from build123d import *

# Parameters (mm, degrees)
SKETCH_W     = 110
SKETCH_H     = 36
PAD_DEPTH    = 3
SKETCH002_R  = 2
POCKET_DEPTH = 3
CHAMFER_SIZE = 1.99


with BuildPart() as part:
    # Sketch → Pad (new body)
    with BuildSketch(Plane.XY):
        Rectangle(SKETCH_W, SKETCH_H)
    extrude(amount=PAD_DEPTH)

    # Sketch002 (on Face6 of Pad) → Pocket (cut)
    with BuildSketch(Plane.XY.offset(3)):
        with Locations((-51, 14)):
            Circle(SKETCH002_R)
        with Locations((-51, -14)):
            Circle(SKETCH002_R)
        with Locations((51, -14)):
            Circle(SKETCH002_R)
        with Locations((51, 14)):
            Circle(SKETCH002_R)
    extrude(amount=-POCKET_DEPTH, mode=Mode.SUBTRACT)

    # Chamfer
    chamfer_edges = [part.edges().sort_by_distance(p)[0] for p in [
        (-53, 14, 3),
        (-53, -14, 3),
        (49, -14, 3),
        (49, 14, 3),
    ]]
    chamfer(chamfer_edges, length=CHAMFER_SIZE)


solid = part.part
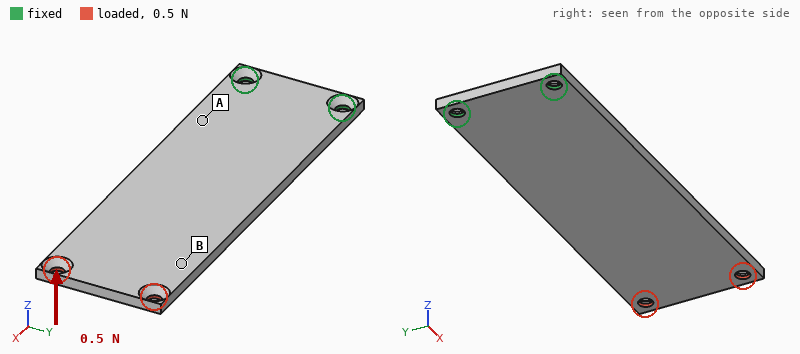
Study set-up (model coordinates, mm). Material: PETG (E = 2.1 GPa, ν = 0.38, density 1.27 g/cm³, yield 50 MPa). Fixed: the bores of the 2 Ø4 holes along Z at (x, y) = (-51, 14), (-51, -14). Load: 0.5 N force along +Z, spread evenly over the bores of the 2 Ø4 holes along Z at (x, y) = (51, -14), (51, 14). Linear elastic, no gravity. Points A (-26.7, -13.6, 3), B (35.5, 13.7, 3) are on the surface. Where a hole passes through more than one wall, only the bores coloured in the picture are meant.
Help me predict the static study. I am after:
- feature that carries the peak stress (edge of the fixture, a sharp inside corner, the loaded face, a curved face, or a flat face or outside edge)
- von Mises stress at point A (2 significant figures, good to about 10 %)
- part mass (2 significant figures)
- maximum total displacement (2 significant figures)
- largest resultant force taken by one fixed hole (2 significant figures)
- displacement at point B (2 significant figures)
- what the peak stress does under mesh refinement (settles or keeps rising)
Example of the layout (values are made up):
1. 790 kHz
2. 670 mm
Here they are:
1. edge of the fixture
2. 0.72 MPa
3. 15 g
4. 1.4 mm
5. 0.39 N
6. 1.0 mm
7. keeps rising
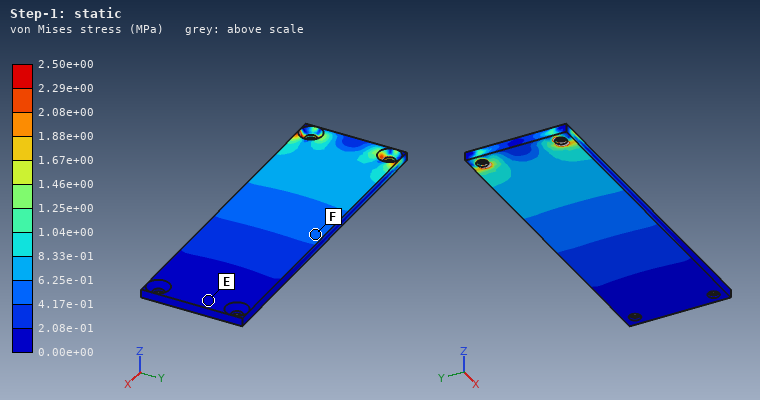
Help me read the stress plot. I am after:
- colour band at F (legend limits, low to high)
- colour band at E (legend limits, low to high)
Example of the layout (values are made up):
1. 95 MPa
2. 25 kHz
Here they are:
1. 4.17e-01 to 6.25e-01 MPa
2. 0.00e+00 to 2.08e-01 MPa
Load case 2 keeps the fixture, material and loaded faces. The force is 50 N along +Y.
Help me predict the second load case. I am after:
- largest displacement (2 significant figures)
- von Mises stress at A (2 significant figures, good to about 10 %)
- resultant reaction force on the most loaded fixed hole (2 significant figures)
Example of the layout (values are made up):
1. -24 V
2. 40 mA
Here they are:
1. 1.2 mm
2. 4.2 MPa
3. 180 N
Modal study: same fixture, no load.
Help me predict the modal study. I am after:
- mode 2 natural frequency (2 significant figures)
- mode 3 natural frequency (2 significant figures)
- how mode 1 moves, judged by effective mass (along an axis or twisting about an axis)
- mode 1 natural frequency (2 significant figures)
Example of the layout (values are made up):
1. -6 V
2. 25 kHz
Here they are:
1. 320 Hz
2. 320 Hz
3. along Z
4. 49 Hz
